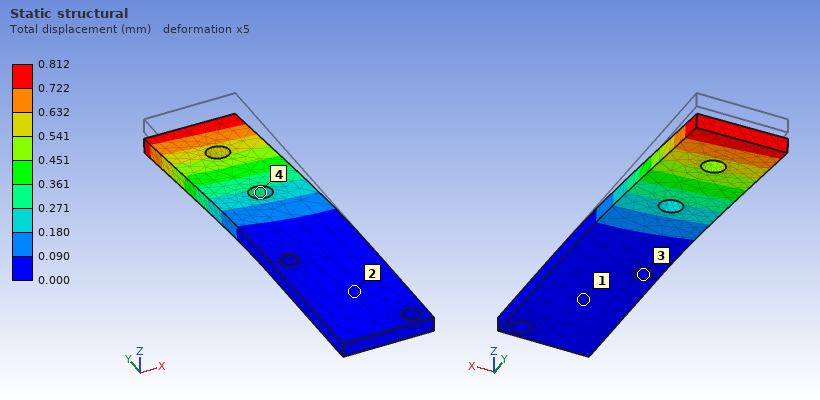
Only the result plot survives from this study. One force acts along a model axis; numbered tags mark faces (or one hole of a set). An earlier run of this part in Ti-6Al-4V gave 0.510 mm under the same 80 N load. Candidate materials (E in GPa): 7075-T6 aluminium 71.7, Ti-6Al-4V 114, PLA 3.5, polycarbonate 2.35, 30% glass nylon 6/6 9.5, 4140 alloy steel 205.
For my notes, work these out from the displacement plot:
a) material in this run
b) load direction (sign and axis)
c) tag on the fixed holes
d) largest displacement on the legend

7075-T6 aluminium
-Z
3
0.812 mm
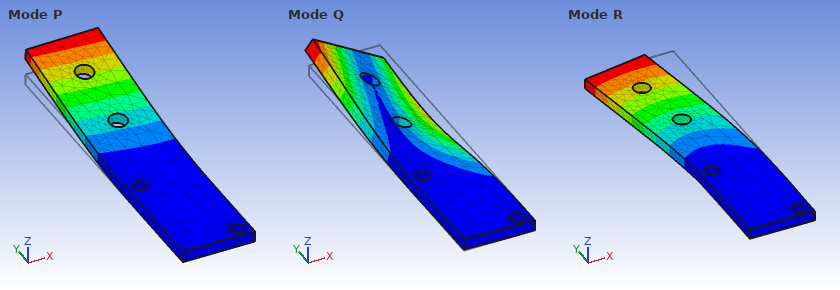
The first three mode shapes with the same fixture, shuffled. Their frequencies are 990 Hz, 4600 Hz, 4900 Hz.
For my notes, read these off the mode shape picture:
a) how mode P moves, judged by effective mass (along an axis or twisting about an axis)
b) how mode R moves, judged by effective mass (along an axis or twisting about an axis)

along Z
along X
